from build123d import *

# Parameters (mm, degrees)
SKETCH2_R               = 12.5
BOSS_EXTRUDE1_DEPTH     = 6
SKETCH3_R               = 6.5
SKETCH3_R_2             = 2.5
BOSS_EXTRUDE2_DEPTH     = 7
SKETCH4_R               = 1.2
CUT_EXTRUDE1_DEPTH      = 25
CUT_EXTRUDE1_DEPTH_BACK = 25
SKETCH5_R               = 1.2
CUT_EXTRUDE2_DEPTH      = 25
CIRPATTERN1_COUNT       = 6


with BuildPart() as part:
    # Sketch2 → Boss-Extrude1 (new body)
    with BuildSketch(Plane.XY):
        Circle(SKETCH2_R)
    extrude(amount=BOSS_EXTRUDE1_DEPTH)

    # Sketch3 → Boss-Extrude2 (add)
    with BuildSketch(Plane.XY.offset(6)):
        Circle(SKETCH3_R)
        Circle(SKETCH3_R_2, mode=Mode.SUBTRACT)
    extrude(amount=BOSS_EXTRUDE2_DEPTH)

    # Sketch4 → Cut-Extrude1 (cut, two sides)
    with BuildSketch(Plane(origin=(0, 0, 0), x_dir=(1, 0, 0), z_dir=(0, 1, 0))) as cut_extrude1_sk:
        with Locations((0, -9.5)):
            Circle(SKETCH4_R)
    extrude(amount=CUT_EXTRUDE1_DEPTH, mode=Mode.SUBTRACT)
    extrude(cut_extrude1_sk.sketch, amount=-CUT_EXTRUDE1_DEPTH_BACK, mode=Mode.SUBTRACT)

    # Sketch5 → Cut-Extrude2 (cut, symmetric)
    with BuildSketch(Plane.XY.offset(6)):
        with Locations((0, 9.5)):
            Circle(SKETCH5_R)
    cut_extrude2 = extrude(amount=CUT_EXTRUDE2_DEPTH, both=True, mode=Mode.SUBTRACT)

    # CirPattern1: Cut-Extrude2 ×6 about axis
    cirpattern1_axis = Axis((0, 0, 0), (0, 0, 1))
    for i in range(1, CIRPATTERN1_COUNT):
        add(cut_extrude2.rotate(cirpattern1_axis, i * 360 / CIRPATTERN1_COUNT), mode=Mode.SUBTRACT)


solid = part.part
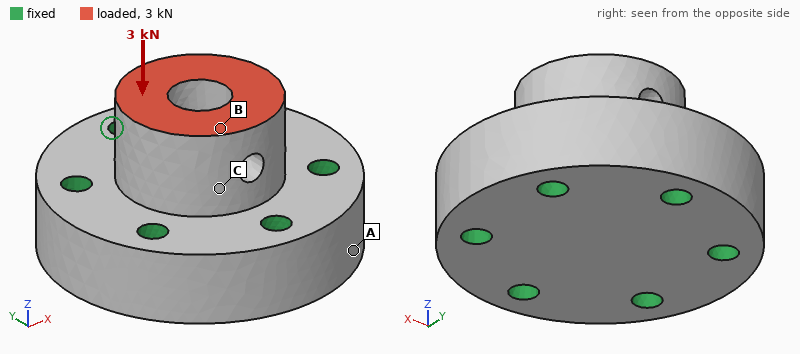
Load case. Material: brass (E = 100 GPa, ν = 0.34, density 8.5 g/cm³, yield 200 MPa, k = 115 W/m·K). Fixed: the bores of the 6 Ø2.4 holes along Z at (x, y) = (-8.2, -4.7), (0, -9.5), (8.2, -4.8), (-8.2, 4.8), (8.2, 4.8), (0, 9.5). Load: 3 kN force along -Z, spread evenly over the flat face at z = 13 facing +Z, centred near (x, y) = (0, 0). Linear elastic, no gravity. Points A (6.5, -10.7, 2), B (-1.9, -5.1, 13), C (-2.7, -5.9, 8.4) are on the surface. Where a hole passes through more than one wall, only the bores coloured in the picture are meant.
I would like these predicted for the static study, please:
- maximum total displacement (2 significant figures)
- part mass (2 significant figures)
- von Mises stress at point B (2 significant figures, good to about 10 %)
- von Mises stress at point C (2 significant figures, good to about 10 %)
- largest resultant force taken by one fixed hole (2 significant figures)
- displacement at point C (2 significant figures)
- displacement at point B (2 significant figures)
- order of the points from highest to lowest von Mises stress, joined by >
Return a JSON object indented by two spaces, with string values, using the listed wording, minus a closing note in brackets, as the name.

{
  "maximum total displacement": "4.7 µm",
  "part mass": "30 g",
  "von Mises stress at point B": "27 MPa",
  "von Mises stress at point C": "37 MPa",
  "largest resultant force taken by one fixed hole": "540 N",
  "displacement at point C": "2.7 µm",
  "displacement at point B": "4.1 µm",
  "order of the points from highest to lowest von Mises stress, joined by >": "C > B > A"
}
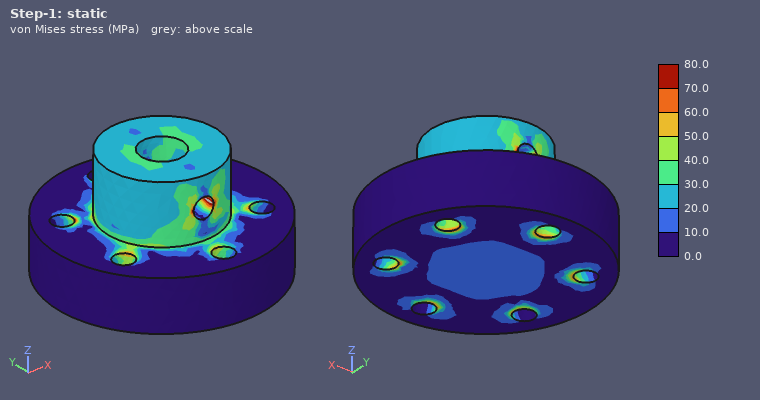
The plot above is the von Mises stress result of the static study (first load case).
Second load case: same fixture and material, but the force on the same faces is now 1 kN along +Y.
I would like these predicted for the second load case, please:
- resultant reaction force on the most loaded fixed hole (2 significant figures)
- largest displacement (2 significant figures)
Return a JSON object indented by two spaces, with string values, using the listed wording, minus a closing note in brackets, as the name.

{
  "resultant reaction force on the most loaded fixed hole": "440 N",
  "largest displacement": "6.7 µm"
}
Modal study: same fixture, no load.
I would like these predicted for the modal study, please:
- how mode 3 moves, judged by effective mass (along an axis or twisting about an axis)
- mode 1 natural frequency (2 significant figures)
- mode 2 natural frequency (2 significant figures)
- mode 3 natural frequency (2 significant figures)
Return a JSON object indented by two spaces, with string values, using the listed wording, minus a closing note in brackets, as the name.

{
  "how mode 3 moves, judged by effective mass": "along Z",
  "mode 1 natural frequency": "40 kHz",
  "mode 2 natural frequency": "41 kHz",
  "mode 3 natural frequency": "51 kHz"
}
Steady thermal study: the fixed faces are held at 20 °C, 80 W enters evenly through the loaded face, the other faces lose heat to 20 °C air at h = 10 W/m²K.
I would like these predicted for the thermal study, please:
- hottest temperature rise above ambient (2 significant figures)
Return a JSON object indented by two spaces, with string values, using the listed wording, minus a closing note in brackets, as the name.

{
  "hottest temperature rise above ambient": "68 K"
}
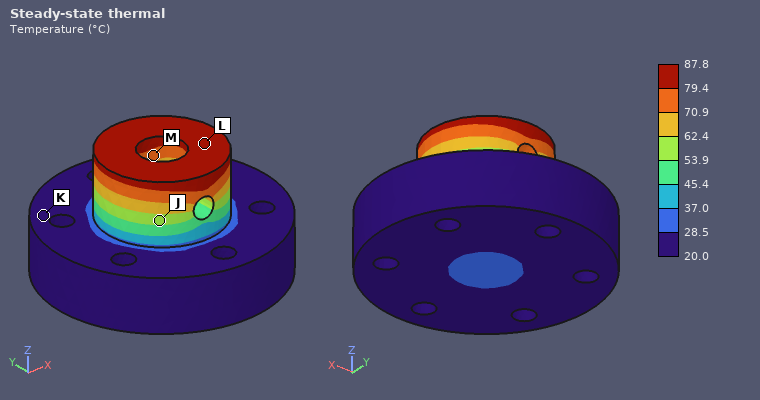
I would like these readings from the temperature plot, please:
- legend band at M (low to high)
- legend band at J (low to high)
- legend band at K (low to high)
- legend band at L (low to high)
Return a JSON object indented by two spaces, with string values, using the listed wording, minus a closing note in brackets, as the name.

{
  "legend band at M": "70.9 to 79.4 °C",
  "legend band at J": "53.9 to 62.4 °C",
  "legend band at K": "20.0 to 28.5 °C",
  "legend band at L": "79.4 to 87.8 °C"
}
